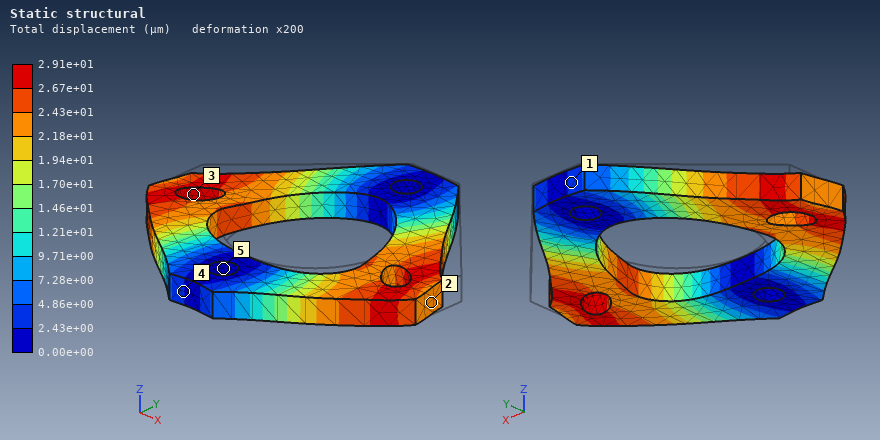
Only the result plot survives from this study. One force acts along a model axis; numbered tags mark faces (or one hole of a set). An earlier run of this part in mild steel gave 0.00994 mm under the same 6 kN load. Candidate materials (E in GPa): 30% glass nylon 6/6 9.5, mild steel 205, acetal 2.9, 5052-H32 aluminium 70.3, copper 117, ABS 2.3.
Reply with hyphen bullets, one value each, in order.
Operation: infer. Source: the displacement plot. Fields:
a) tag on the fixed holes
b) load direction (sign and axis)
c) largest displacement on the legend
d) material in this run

- 5
- -Y
- 2.91e+01 µm
- 5052-H32 aluminium
